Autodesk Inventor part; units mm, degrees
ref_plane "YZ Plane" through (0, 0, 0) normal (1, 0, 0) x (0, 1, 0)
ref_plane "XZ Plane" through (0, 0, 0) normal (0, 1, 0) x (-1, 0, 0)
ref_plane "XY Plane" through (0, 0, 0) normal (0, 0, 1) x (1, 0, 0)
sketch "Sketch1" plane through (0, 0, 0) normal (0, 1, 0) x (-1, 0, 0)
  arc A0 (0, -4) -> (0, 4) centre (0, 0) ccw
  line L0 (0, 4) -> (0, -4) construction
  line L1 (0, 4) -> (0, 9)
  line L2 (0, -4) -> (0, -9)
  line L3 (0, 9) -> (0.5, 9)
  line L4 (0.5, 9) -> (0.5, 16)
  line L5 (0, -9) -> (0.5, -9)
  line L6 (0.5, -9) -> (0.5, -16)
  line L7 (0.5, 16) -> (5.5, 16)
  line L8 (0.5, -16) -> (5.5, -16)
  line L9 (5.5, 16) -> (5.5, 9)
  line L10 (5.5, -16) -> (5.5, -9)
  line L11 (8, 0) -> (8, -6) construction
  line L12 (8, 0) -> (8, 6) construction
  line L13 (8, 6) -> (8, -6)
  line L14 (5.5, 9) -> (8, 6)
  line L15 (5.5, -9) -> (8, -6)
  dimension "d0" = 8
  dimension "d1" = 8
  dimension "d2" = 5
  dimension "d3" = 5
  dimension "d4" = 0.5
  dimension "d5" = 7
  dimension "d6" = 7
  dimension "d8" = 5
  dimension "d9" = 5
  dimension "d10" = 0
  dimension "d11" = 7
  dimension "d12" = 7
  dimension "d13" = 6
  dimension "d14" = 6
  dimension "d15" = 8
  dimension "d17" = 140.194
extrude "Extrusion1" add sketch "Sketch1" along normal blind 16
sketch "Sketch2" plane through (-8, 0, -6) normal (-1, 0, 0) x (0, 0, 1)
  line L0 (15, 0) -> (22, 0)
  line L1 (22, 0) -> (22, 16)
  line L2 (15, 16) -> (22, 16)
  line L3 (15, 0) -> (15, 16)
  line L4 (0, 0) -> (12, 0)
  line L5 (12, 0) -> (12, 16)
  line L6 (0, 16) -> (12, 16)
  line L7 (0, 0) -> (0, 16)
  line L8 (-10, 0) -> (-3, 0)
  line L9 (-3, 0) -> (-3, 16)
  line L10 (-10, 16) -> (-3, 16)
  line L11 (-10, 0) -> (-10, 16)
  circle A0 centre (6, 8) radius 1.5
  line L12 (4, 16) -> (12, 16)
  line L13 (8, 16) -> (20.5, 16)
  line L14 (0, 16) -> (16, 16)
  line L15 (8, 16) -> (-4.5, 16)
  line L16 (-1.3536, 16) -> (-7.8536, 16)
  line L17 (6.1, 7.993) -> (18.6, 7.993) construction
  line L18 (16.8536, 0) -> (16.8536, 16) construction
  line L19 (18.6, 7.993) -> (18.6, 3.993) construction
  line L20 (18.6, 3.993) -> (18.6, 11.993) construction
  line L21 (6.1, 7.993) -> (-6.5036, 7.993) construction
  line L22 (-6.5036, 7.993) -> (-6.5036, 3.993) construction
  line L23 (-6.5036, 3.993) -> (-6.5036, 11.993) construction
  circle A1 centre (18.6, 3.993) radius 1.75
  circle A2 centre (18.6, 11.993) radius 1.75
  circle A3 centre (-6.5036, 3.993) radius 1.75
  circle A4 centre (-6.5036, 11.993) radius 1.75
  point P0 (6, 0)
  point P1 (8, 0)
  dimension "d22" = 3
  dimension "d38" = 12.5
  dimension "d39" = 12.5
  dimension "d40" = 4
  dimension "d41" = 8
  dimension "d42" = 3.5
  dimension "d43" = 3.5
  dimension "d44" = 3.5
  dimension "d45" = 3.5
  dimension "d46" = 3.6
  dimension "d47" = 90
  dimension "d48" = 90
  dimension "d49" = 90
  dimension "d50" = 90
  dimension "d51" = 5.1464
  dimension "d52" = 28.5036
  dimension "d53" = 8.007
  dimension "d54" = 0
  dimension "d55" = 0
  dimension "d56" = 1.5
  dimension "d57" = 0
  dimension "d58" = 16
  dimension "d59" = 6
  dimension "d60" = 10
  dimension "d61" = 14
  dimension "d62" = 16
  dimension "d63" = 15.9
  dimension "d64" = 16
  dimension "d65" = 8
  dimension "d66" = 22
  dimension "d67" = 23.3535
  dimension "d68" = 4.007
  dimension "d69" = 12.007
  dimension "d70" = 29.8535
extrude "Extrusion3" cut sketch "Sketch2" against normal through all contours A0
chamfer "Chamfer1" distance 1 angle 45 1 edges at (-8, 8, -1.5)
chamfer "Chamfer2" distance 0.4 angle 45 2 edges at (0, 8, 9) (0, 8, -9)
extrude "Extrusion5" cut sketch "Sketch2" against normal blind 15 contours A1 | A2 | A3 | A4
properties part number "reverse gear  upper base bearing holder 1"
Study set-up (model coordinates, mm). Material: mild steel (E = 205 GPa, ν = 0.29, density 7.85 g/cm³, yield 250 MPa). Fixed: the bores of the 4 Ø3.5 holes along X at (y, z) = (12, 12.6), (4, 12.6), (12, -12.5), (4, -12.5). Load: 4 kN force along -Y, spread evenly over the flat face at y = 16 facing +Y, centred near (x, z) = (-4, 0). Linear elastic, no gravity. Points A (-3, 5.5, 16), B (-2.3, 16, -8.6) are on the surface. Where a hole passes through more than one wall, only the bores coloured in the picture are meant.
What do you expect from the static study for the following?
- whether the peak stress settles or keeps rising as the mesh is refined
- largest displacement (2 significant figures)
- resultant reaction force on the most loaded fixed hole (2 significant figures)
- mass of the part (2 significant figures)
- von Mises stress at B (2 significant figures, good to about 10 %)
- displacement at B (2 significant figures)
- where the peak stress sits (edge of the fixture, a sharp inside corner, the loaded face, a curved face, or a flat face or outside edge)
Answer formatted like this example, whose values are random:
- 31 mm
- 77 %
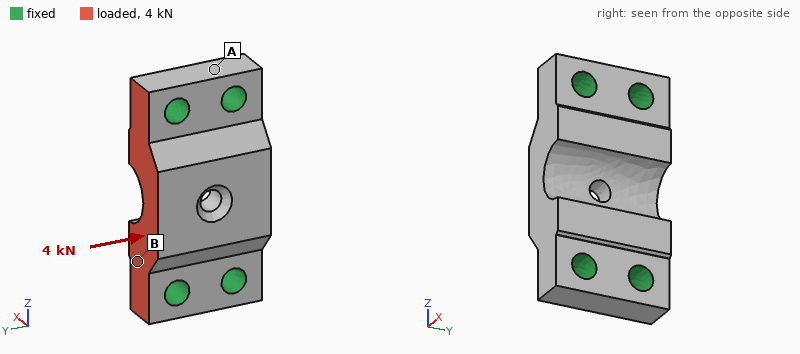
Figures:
- keeps rising
- 3.6 µm
- 1.4 kN
- 21 g
- 27 MPa
- 1.6 µm
- edge of the fixture
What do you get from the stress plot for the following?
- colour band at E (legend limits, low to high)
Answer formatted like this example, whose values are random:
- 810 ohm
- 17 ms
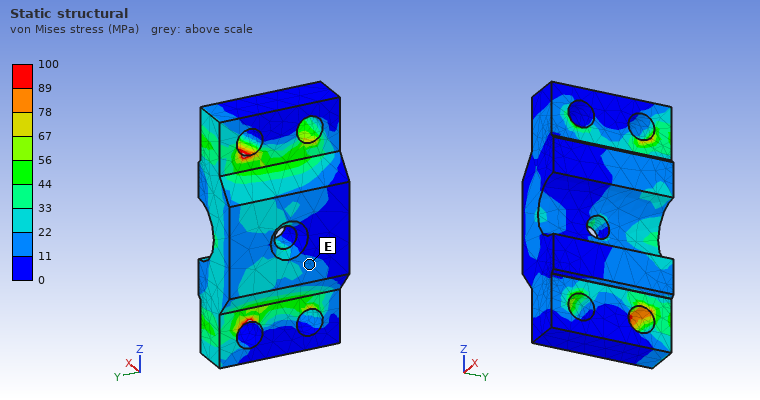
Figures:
- 11 to 22 MPa
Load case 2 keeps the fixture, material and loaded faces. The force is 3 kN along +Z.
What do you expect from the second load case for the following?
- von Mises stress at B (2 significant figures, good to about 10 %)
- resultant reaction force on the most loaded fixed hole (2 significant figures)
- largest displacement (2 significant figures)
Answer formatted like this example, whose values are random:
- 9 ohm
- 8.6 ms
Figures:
- 36 MPa
- 1.4 kN
- 1.9 µm
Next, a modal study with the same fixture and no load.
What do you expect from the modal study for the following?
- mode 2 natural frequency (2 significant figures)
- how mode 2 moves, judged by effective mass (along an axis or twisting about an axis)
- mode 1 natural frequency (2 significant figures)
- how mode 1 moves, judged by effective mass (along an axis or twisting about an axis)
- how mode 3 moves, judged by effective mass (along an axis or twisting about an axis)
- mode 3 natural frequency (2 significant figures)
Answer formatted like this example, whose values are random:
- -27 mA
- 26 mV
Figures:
- 44 kHz
- along Y
- 41 kHz
- along X
- along Y
- 63 kHz
